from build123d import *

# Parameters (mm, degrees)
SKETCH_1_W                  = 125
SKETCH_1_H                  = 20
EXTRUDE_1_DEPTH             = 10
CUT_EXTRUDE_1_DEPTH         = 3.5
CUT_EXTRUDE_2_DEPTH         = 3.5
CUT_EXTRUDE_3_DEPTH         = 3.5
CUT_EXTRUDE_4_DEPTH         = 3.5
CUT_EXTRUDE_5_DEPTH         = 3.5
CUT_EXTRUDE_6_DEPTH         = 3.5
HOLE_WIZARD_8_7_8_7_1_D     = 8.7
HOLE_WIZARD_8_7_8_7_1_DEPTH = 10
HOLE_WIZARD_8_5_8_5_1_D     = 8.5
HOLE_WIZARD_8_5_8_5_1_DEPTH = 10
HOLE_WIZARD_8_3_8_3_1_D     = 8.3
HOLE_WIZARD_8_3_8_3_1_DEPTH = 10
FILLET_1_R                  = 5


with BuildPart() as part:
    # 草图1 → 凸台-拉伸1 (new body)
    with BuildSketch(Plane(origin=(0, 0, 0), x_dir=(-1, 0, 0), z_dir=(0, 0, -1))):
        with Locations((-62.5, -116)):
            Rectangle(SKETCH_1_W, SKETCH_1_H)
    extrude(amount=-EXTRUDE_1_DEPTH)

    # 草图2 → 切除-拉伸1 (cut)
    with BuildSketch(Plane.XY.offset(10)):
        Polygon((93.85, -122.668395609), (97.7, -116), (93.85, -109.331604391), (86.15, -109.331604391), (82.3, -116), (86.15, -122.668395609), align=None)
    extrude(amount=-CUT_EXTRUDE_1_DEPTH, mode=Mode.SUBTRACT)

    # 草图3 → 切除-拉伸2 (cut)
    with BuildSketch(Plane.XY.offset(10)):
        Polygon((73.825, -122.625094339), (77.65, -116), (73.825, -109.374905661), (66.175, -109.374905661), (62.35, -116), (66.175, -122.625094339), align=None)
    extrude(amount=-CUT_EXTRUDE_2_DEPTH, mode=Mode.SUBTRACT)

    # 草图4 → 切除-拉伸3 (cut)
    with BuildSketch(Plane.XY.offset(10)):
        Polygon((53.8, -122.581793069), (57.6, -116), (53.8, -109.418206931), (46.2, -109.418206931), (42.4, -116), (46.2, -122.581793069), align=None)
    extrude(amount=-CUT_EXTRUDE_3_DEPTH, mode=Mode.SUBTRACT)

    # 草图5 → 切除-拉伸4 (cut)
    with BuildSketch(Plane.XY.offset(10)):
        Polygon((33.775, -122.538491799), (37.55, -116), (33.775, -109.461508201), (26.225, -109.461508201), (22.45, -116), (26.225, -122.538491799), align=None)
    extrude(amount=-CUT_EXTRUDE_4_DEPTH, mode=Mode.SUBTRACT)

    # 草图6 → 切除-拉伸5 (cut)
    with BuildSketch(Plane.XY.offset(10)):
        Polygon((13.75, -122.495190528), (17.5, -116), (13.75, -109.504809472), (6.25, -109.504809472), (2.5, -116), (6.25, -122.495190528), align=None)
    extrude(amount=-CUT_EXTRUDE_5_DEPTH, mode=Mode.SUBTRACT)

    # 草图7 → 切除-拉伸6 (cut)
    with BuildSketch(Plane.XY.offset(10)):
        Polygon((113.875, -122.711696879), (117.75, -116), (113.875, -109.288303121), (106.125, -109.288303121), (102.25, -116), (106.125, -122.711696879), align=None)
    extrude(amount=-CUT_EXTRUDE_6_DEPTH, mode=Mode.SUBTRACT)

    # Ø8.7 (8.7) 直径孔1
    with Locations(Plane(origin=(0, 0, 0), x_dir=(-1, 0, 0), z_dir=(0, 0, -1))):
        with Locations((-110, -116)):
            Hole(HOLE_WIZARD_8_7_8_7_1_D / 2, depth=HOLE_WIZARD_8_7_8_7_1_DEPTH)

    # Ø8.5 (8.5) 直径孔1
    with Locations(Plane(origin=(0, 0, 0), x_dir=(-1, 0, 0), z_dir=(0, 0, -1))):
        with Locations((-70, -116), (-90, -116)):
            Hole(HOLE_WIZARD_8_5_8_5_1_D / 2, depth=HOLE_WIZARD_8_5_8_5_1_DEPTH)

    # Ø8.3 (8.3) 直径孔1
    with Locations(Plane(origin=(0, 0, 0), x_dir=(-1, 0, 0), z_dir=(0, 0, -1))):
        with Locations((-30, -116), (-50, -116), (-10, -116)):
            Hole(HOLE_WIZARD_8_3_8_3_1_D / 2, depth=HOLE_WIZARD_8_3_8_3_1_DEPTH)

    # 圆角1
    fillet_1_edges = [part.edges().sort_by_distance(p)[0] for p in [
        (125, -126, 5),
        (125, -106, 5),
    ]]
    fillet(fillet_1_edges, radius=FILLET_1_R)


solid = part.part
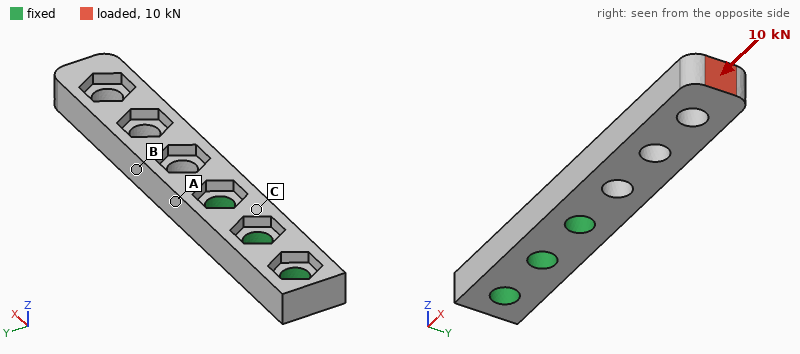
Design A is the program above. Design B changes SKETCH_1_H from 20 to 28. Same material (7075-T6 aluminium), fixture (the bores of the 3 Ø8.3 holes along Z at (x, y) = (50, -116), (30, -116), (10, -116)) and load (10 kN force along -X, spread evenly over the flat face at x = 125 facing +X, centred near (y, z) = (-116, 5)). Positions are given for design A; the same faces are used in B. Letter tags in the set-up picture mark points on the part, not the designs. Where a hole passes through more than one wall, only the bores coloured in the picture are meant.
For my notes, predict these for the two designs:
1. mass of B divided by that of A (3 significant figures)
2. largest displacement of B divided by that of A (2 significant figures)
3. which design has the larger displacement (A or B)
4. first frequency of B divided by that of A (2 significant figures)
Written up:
1.51
0.46
A
1.0
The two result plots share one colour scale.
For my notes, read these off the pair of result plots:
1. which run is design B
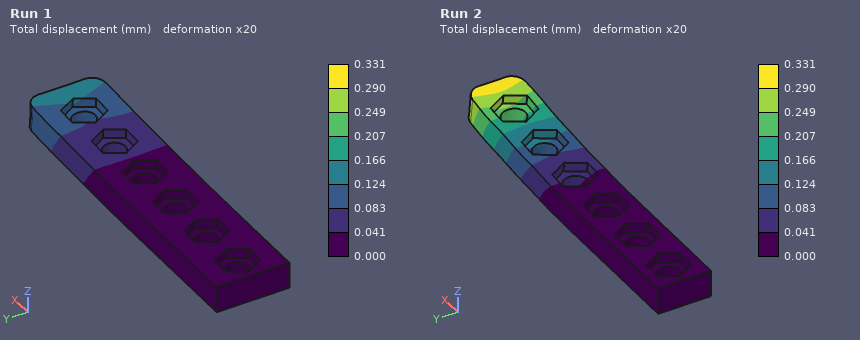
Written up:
Run 1
